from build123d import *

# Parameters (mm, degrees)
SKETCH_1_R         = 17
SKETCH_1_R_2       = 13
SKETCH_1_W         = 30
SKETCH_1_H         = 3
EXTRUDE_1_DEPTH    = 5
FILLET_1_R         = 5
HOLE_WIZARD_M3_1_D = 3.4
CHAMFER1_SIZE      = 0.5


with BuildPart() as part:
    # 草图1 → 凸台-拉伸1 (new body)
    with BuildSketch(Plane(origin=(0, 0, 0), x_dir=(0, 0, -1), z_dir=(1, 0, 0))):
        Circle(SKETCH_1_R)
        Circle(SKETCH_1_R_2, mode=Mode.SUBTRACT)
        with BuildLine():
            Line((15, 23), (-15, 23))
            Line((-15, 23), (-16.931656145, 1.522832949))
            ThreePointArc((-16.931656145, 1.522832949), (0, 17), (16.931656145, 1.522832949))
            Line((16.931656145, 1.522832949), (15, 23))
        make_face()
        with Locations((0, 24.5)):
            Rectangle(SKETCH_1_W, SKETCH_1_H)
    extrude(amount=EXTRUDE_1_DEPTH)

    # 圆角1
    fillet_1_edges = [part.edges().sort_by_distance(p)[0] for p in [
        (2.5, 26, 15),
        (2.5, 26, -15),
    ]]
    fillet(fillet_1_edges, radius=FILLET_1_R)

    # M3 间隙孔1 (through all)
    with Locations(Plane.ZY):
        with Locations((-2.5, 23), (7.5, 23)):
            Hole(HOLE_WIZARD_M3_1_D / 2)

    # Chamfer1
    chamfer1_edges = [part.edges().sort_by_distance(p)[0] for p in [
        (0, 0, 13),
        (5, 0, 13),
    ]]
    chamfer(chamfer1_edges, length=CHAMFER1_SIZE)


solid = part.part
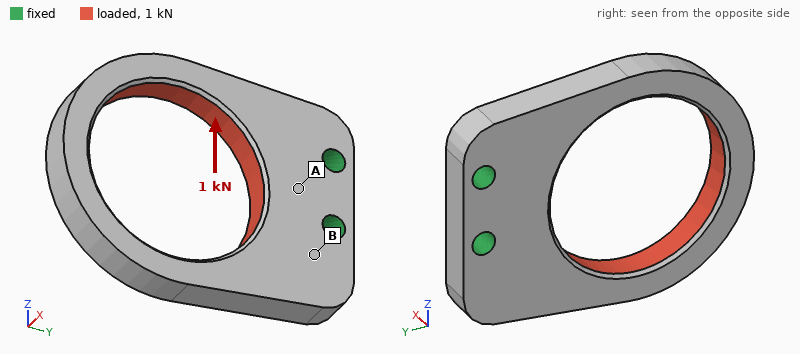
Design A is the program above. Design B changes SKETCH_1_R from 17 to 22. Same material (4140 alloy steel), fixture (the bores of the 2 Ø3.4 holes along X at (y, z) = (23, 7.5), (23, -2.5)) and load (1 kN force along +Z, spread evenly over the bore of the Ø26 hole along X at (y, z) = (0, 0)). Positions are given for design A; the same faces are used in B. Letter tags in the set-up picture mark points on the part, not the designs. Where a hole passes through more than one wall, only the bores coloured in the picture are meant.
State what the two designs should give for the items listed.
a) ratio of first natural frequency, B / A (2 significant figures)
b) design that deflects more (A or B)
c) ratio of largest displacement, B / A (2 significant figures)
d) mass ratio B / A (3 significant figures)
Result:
0.64
A
0.61
1.58
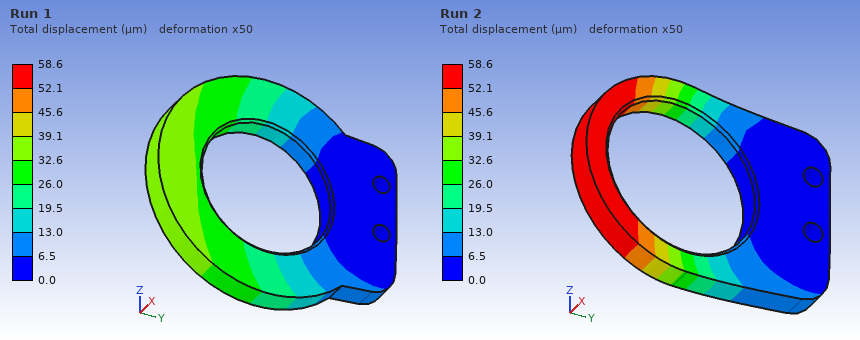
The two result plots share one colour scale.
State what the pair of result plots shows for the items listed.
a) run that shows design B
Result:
Run 1
